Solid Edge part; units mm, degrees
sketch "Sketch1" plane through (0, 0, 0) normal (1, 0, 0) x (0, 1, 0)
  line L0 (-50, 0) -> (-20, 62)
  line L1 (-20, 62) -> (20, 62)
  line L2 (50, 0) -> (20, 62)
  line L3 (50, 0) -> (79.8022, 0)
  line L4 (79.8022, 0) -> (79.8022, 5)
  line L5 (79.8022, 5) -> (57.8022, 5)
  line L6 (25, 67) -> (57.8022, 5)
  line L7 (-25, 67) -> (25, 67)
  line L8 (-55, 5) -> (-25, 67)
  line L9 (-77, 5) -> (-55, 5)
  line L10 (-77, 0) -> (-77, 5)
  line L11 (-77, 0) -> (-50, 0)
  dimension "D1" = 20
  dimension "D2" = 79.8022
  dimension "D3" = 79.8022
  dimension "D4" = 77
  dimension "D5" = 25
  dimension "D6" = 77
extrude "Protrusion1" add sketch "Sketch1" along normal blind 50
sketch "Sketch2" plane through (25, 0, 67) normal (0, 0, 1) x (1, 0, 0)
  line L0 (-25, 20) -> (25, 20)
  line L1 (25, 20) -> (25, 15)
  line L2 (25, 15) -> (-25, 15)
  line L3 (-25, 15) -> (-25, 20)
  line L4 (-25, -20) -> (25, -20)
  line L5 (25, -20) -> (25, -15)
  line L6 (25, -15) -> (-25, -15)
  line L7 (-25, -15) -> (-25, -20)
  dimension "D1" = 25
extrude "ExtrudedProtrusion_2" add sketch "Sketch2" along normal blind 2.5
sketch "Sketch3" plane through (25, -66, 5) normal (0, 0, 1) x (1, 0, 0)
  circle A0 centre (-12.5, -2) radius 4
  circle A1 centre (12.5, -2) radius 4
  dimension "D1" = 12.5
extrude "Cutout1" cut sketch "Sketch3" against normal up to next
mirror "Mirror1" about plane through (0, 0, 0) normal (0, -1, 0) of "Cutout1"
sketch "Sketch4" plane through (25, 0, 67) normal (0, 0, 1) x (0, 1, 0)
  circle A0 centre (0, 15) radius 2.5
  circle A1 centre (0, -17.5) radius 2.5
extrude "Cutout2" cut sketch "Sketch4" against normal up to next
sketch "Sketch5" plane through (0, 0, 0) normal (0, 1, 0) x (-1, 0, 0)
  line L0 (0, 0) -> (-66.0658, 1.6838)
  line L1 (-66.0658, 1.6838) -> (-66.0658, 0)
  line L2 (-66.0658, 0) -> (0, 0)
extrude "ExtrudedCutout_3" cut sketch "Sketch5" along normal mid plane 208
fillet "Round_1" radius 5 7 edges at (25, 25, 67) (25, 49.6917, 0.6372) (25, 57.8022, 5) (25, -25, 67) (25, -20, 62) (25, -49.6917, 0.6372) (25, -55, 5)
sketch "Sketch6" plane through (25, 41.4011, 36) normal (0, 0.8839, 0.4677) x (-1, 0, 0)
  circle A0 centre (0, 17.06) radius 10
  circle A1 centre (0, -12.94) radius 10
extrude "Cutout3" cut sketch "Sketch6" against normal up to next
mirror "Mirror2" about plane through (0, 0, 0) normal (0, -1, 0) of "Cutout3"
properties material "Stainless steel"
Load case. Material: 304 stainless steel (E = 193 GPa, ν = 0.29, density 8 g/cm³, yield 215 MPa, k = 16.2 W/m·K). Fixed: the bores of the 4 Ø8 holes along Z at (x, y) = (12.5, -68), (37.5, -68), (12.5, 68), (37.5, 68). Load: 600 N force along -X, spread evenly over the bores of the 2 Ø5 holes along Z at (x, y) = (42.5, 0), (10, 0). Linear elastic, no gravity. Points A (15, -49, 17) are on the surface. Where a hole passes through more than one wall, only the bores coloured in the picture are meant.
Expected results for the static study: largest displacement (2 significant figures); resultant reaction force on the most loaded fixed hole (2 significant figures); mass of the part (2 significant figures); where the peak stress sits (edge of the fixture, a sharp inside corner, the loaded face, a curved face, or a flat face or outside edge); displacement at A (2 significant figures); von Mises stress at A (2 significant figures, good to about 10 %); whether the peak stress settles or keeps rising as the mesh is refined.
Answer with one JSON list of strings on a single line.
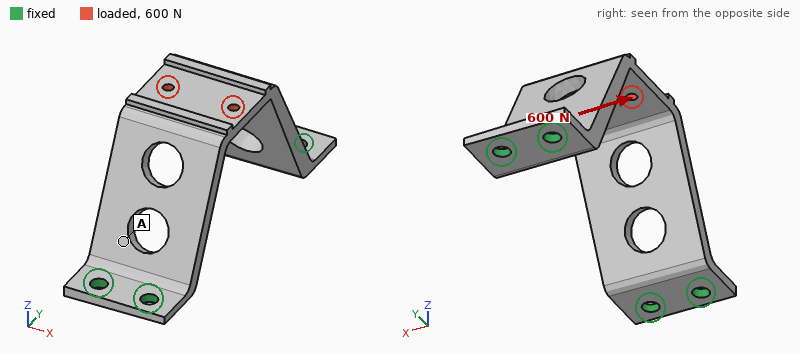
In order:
["32 µm", "930 N", "510 g", "edge of the fixture", "7.1 µm", "6.9 MPa", "keeps rising"]
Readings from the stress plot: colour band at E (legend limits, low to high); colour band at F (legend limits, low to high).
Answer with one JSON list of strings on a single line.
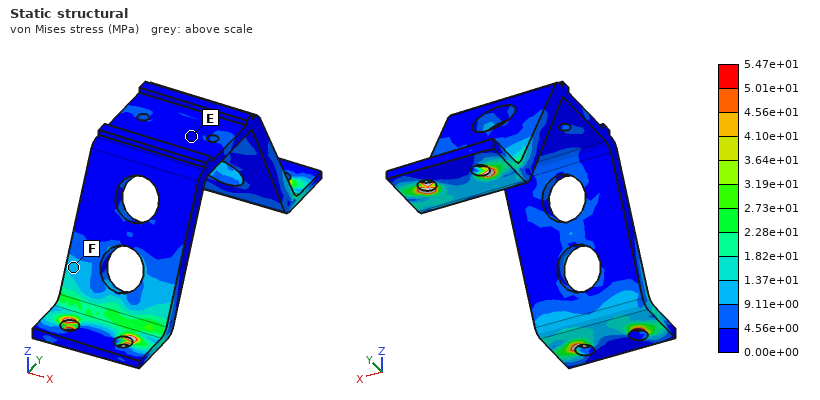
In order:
["0.00e+00 to 4.56e+00 MPa", "9.11e+00 to 1.37e+01 MPa"]
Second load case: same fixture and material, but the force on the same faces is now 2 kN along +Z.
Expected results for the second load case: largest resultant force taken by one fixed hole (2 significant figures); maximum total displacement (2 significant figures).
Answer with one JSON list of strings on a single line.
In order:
["690 N", "30 µm"]
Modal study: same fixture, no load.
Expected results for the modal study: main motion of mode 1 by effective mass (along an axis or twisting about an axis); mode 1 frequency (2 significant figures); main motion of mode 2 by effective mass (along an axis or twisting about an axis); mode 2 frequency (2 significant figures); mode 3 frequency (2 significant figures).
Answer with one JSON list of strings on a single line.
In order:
["along Y", "1500 Hz", "along X", "1600 Hz", "2400 Hz"]
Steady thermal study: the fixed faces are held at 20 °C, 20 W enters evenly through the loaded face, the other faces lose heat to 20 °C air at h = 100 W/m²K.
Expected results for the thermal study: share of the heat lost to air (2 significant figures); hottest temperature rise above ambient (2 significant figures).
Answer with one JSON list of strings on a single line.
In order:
["99 %", "64 K"]
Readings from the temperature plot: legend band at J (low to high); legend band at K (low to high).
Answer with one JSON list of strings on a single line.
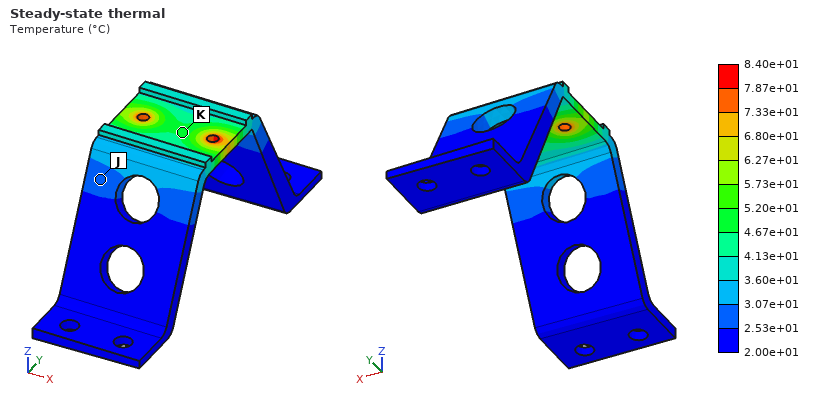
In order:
["2.53e+01 to 3.07e+01 °C", "4.67e+01 to 5.20e+01 °C"]
